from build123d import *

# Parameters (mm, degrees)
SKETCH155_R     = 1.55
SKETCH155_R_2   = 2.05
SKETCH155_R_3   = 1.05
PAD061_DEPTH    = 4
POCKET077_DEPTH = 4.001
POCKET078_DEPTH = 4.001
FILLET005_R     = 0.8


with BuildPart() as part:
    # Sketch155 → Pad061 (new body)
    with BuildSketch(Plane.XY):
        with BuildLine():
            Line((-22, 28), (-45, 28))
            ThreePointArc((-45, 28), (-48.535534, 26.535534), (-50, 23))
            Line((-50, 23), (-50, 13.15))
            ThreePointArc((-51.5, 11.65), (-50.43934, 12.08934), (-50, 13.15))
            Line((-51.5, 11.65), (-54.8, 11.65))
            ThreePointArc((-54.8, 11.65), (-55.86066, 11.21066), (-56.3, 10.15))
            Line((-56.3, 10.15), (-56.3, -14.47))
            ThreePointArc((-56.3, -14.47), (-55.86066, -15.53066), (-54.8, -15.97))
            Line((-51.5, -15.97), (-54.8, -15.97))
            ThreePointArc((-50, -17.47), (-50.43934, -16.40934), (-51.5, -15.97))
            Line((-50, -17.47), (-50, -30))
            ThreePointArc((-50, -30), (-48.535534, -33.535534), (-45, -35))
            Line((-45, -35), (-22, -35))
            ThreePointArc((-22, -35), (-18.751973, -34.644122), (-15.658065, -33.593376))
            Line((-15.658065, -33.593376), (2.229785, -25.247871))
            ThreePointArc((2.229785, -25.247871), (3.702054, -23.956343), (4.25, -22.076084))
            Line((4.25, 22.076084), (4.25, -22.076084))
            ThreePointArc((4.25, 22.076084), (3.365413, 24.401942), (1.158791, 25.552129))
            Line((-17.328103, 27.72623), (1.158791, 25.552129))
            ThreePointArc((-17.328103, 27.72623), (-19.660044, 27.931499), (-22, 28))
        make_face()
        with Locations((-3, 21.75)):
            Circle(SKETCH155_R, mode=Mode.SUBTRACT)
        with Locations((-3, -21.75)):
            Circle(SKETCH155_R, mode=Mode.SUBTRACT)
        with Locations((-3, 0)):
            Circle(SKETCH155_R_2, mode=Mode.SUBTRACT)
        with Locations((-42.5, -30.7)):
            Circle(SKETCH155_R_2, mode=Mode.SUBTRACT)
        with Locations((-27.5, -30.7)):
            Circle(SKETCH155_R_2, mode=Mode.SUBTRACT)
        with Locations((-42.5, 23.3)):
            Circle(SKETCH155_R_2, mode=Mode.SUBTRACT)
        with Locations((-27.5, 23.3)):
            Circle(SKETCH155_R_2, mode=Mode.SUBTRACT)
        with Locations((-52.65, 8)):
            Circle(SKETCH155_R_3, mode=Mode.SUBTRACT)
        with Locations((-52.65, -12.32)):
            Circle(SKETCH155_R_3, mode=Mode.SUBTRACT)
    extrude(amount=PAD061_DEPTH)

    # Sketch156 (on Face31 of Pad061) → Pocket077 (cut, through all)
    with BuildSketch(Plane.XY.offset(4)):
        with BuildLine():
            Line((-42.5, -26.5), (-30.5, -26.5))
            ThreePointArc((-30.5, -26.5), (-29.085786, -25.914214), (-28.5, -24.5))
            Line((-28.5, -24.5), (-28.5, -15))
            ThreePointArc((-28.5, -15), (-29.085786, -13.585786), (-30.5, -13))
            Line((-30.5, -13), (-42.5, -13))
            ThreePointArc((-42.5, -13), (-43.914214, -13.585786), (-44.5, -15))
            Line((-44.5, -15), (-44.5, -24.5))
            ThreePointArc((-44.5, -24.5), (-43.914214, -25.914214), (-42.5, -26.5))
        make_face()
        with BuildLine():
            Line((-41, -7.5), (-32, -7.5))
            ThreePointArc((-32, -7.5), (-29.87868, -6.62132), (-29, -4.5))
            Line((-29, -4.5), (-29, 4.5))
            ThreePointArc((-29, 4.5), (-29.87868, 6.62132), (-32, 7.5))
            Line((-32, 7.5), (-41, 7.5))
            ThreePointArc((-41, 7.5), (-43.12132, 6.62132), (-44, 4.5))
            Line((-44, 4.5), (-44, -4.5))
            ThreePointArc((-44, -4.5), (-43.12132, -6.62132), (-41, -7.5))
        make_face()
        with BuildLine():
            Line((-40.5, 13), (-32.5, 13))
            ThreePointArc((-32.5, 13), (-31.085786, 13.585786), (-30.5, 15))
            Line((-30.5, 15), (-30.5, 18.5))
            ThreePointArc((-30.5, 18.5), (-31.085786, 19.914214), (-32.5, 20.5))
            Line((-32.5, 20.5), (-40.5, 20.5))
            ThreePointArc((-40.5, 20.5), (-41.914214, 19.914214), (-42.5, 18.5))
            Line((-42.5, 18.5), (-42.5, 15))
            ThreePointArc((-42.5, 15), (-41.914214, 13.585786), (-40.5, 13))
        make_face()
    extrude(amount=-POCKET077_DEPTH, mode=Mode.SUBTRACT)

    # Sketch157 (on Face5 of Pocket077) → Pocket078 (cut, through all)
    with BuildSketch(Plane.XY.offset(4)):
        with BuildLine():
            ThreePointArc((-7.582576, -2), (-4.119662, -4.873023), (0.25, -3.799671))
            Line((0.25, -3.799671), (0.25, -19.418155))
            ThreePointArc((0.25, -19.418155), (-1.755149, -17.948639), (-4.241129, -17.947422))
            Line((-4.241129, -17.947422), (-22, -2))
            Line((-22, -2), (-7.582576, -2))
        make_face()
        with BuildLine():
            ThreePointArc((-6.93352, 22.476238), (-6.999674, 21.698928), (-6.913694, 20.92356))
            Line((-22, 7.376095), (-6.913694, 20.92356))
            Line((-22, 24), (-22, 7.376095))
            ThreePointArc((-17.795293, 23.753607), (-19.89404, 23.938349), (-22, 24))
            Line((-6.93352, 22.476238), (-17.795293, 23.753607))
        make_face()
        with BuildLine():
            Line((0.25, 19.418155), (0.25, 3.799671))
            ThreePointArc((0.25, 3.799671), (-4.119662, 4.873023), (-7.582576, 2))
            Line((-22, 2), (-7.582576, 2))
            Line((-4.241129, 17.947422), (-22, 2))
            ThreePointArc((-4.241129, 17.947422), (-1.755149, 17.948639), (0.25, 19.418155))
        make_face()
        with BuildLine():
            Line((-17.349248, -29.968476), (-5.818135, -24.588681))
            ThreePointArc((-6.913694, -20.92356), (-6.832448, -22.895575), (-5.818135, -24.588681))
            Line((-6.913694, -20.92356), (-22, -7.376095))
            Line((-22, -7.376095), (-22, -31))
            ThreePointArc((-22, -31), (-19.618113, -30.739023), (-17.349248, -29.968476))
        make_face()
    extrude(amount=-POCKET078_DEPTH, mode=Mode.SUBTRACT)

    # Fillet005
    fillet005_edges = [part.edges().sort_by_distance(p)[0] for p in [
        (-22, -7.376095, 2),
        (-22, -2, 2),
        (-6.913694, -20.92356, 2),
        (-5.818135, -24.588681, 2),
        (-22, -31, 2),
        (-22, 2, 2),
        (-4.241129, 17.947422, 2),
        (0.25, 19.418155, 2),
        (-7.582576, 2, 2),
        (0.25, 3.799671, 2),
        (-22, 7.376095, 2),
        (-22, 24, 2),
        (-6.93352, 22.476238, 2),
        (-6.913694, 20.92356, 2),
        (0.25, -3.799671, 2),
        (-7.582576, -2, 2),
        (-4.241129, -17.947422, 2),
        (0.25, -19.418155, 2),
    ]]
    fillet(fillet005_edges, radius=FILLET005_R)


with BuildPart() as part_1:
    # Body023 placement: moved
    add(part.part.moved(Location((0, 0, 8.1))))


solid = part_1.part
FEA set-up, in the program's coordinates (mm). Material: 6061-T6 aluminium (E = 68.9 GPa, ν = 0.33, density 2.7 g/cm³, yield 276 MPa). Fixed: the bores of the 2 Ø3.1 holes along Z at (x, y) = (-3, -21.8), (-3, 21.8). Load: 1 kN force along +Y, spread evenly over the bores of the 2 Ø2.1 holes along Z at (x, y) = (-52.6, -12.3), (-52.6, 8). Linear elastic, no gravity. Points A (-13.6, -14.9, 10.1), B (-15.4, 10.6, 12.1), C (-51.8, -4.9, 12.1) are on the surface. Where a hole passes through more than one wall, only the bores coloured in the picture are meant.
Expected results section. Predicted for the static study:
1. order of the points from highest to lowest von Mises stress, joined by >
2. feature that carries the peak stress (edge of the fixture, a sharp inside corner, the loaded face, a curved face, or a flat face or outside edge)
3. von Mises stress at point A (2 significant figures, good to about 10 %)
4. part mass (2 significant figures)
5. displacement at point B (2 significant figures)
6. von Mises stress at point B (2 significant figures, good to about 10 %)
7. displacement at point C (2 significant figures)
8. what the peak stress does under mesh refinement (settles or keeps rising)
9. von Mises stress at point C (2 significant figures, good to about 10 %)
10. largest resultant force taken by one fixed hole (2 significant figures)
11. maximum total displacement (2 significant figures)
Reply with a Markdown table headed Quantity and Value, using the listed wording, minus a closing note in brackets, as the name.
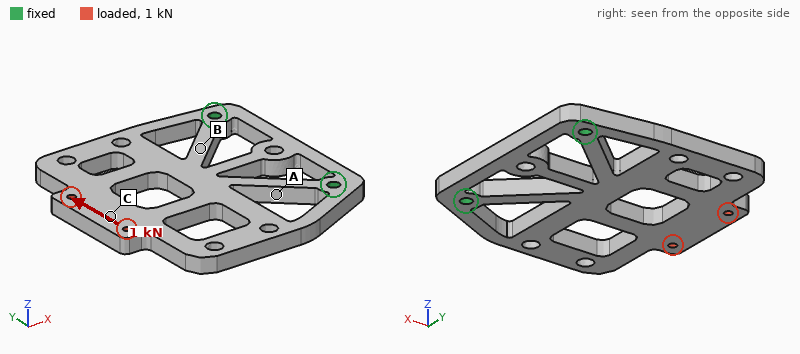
| Quantity | Value |
|---|---|
| order of the points from highest to lowest von Mises stress, joined by > | A > B > C |
| feature that carries the peak stress | a sharp inside corner |
| von Mises stress at point A | 65 MPa |
| part mass | 22 g |
| displacement at point B | 16 µm |
| von Mises stress at point B | 43 MPa |
| displacement at point C | 84 µm |
| what the peak stress does under mesh refinement | keeps rising |
| von Mises stress at point C | 14 MPa |
| largest resultant force taken by one fixed hole | 1.2 kN |
| maximum total displacement | 90 µm |
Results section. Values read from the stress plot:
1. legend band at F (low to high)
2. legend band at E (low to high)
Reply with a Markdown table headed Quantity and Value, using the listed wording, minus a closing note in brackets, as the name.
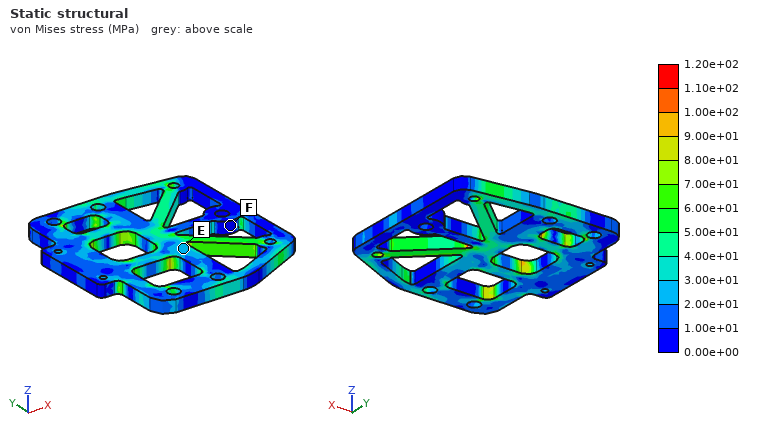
| Quantity | Value |
|---|---|
| legend band at F | 0.00e+00 to 1.00e+01 MPa |
| legend band at E | 2.00e+01 to 3.00e+01 MPa |
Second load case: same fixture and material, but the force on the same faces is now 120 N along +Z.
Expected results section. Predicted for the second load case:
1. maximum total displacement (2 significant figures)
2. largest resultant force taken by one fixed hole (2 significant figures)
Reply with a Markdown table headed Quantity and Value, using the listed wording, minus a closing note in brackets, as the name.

| Quantity | Value |
|---|---|
| maximum total displacement | 0.90 mm |
| largest resultant force taken by one fixed hole | 62 N |
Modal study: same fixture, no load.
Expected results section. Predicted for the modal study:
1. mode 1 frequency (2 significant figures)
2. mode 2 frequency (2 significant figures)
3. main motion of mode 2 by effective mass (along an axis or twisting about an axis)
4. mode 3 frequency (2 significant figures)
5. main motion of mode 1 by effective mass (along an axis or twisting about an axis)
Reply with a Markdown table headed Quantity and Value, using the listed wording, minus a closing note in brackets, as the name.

| Quantity | Value |
|---|---|
| mode 1 frequency | 770 Hz |
| mode 2 frequency | 2000 Hz |
| main motion of mode 2 by effective mass | twisting about X |
| mode 3 frequency | 4700 Hz |
| main motion of mode 1 by effective mass | along Z |
